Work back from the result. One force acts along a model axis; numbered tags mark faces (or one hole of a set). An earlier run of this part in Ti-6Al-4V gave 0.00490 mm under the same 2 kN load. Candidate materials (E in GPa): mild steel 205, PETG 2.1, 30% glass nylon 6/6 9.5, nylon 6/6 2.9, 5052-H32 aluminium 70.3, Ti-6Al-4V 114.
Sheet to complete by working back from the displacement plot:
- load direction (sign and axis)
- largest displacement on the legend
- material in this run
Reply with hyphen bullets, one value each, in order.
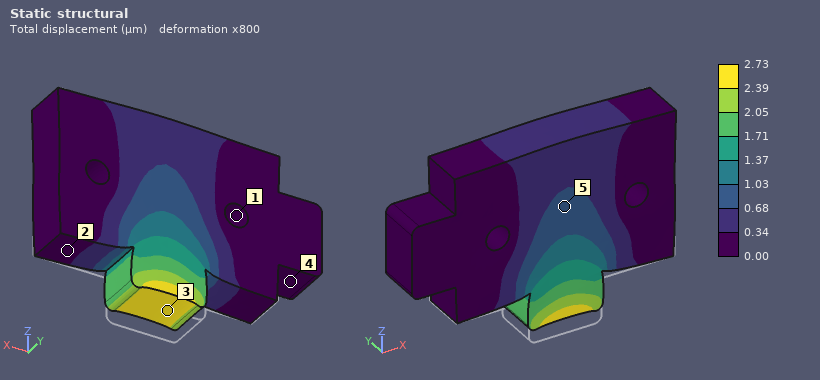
- +Z
- 2.73 µm
- mild steel
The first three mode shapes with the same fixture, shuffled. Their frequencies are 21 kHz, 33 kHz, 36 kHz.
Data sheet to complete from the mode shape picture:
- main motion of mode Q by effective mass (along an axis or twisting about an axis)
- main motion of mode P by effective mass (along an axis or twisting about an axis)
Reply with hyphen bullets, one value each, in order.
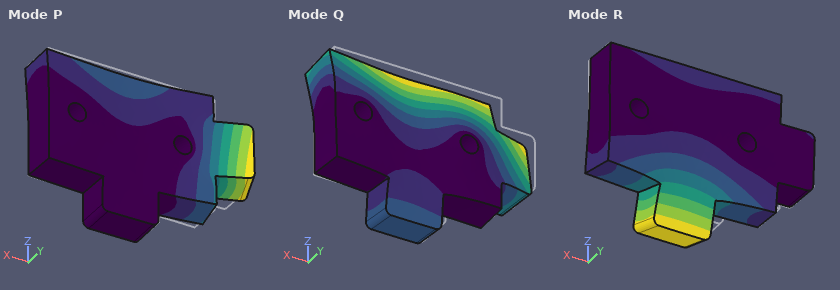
- along Y
- twisting about Z
